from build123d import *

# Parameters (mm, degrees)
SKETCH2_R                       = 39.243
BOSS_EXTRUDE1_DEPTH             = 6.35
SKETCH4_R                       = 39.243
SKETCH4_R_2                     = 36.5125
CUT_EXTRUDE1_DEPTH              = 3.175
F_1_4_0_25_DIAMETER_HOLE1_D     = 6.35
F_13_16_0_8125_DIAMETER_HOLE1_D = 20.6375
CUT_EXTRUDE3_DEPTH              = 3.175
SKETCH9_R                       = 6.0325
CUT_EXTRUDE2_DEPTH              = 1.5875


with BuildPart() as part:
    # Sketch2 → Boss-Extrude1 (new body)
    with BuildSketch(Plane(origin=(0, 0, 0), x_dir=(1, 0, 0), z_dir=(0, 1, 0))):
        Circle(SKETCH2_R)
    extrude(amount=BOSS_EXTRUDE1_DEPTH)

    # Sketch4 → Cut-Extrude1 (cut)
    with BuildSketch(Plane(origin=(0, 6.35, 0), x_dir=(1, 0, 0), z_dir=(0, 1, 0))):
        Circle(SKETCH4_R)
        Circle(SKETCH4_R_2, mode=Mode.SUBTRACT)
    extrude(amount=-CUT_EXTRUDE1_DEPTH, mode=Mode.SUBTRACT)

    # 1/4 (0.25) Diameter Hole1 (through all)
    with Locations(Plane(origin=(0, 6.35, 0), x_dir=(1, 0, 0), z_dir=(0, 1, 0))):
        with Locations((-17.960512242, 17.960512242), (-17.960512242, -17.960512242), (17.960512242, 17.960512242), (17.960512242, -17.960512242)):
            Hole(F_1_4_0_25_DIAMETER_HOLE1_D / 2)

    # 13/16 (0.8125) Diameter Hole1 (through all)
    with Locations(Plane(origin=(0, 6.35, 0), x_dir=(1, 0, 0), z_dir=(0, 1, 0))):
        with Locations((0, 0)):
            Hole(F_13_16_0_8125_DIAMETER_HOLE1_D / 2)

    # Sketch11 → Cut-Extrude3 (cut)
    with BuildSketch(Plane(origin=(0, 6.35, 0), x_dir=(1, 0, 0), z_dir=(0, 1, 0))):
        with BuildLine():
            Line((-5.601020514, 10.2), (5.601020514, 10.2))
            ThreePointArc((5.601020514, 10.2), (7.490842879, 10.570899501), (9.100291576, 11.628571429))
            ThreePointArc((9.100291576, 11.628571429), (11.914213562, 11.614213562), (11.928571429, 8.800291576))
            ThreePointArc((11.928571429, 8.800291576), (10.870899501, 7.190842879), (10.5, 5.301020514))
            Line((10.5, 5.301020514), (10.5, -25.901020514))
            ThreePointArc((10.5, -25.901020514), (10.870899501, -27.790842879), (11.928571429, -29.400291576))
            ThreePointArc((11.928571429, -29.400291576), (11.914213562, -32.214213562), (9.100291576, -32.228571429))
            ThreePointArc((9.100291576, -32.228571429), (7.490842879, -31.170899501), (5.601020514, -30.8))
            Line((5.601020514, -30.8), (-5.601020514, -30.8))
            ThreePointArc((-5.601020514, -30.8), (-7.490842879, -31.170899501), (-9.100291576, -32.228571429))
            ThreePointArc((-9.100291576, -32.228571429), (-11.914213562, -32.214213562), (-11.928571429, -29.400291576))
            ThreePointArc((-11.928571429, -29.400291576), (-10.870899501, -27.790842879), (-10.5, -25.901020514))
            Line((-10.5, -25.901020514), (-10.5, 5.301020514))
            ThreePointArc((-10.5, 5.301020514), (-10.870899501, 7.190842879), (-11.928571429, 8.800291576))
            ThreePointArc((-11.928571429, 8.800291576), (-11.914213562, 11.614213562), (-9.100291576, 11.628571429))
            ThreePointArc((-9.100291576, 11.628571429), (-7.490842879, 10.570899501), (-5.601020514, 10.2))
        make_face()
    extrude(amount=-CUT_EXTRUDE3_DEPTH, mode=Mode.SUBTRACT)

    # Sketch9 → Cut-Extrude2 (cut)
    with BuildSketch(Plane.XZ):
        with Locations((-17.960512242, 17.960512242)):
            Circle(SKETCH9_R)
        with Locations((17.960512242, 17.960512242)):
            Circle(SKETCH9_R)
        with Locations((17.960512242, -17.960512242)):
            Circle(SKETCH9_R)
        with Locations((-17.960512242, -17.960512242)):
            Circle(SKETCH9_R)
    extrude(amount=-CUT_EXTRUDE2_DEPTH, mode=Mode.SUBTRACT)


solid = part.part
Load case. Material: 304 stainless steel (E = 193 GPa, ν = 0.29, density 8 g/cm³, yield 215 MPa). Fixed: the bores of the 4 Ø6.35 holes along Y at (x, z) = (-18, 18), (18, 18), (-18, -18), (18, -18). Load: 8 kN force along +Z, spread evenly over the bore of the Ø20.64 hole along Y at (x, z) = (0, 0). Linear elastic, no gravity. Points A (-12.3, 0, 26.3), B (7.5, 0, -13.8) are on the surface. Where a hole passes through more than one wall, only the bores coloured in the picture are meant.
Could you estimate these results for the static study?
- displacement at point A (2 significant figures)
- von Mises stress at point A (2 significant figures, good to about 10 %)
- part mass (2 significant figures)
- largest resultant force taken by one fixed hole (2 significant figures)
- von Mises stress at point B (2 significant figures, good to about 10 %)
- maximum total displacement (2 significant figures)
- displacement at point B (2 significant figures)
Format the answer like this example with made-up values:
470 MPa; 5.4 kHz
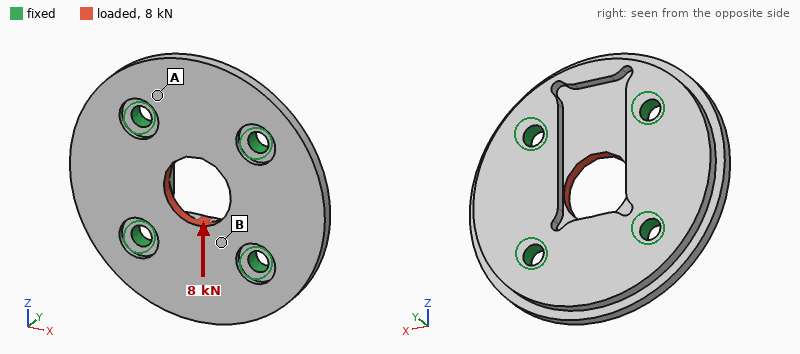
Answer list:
1.7 µm; 13 MPa; 190 g; 2.1 kN; 33 MPa; 4.5 µm; 2.5 µm
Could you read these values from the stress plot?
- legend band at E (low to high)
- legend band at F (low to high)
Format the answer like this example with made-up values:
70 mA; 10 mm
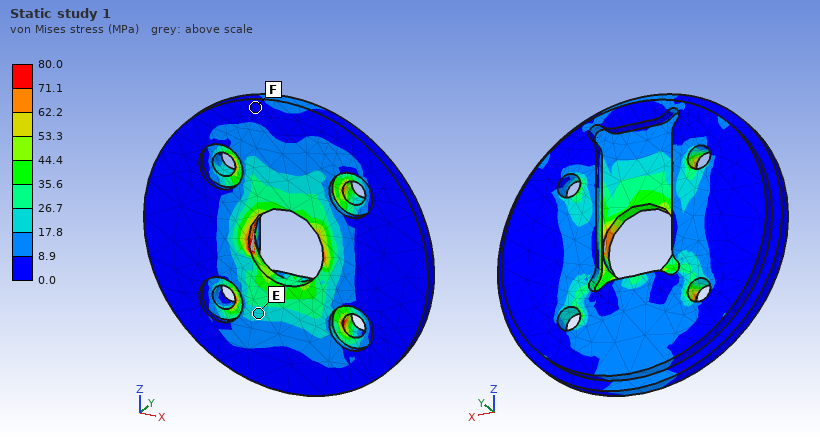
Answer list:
17.8 to 26.7 MPa; 0.0 to 8.9 MPa
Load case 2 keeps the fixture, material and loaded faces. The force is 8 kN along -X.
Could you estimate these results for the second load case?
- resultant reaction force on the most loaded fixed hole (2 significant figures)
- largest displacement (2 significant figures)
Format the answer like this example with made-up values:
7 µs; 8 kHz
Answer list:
2.2 kN; 5.5 µm
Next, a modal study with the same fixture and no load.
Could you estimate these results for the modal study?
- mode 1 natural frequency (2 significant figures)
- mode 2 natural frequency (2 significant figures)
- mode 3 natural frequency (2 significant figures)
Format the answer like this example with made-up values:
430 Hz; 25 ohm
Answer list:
9800 Hz; 11 kHz; 11 kHz
